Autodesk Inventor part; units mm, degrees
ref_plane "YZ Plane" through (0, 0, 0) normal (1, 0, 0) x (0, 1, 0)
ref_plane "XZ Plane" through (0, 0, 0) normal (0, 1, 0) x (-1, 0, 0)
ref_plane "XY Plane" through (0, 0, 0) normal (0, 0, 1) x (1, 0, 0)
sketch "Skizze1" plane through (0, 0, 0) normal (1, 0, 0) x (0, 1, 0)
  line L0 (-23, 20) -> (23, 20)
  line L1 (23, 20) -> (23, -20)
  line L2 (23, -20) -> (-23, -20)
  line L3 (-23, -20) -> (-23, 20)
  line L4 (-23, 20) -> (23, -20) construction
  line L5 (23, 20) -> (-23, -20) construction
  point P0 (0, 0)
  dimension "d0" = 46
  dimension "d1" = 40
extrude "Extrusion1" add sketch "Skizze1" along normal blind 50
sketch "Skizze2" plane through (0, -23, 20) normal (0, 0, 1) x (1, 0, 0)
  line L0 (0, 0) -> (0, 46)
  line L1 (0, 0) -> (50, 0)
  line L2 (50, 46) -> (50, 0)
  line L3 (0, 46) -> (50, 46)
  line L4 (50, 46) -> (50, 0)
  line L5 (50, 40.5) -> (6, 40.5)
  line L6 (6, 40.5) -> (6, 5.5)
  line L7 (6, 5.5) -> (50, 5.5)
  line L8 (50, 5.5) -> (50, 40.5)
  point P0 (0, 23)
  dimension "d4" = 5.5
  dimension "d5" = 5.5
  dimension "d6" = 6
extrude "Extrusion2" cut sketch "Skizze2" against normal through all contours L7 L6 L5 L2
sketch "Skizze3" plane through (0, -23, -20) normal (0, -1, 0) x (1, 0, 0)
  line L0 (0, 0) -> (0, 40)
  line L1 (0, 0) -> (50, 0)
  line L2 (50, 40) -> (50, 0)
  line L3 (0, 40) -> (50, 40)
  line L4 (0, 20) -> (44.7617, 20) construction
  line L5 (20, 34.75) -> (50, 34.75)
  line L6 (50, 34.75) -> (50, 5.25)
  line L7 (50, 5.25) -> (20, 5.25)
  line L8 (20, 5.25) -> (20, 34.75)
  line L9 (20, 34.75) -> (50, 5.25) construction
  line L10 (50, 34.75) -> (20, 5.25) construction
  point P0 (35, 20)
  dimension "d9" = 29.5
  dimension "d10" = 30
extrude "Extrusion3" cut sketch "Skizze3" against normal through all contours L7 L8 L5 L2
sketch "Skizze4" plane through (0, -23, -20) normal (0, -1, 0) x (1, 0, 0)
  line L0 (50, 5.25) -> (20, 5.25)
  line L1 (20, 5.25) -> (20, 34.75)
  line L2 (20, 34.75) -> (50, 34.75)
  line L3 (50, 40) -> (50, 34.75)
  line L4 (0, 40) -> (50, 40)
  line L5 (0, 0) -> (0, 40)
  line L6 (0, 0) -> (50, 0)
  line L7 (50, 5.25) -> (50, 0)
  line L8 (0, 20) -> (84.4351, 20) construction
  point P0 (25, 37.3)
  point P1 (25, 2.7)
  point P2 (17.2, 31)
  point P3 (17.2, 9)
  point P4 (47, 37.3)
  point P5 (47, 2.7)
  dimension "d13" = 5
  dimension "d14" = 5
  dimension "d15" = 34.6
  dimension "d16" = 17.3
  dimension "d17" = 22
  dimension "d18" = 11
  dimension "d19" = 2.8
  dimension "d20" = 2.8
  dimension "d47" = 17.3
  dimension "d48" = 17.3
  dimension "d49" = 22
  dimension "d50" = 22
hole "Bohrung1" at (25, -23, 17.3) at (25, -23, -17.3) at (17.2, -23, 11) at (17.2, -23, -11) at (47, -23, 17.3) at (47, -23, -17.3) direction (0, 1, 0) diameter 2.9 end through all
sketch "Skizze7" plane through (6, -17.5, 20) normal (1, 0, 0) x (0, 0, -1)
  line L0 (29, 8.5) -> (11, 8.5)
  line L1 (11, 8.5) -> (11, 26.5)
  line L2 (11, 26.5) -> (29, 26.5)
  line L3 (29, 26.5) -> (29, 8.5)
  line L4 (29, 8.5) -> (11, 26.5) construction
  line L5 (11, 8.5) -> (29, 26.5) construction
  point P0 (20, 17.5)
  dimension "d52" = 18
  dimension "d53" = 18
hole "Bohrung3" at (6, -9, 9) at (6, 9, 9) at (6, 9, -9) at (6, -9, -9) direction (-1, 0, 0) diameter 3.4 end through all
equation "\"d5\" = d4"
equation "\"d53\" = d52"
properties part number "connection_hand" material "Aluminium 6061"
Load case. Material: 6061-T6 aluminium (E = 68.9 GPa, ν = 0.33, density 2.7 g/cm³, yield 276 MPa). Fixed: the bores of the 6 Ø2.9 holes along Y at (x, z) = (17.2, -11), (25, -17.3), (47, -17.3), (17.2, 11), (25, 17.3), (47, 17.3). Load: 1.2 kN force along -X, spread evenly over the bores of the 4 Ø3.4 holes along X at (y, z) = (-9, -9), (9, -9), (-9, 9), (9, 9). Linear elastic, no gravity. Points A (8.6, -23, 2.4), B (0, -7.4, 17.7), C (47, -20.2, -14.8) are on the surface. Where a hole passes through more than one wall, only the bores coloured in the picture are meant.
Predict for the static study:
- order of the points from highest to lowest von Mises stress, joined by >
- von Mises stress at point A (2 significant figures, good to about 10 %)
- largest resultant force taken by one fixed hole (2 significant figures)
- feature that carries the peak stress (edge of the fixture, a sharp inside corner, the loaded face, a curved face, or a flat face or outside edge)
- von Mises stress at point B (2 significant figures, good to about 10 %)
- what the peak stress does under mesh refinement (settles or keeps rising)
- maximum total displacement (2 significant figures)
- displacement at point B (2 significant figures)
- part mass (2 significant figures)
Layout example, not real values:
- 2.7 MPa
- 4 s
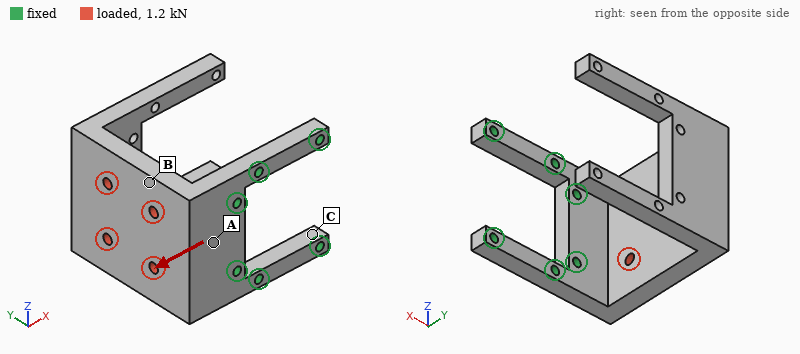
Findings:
- A > B > C
- 93 MPa
- 650 N
- edge of the fixture
- 49 MPa
- keeps rising
- 0.84 mm
- 0.19 mm
- 54 g
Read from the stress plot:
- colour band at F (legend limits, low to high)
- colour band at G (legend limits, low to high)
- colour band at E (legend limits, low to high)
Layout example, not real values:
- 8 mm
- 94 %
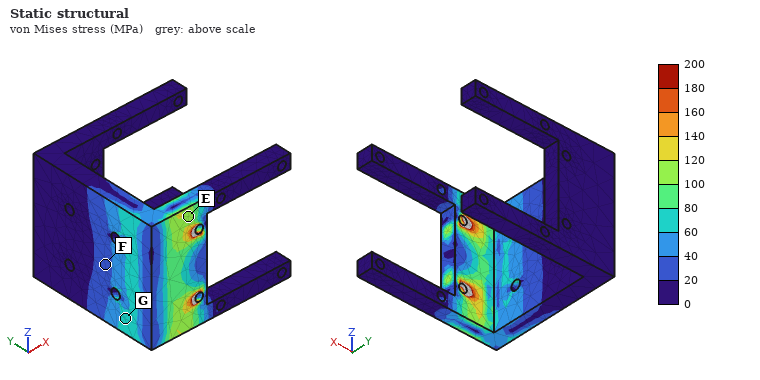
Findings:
- 20 to 40 MPa
- 60 to 80 MPa
- 100 to 120 MPa
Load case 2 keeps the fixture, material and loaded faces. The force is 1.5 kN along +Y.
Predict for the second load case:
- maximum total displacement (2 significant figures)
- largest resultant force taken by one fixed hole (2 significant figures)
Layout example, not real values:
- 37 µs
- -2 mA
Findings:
- 0.28 mm
- 950 N
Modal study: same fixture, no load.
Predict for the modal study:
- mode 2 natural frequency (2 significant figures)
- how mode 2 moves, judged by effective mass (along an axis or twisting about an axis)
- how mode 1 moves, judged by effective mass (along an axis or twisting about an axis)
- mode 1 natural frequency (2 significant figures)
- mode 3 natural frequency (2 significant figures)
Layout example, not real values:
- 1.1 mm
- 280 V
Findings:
- 1700 Hz
- along Z
- along X
- 960 Hz
- 2500 Hz
